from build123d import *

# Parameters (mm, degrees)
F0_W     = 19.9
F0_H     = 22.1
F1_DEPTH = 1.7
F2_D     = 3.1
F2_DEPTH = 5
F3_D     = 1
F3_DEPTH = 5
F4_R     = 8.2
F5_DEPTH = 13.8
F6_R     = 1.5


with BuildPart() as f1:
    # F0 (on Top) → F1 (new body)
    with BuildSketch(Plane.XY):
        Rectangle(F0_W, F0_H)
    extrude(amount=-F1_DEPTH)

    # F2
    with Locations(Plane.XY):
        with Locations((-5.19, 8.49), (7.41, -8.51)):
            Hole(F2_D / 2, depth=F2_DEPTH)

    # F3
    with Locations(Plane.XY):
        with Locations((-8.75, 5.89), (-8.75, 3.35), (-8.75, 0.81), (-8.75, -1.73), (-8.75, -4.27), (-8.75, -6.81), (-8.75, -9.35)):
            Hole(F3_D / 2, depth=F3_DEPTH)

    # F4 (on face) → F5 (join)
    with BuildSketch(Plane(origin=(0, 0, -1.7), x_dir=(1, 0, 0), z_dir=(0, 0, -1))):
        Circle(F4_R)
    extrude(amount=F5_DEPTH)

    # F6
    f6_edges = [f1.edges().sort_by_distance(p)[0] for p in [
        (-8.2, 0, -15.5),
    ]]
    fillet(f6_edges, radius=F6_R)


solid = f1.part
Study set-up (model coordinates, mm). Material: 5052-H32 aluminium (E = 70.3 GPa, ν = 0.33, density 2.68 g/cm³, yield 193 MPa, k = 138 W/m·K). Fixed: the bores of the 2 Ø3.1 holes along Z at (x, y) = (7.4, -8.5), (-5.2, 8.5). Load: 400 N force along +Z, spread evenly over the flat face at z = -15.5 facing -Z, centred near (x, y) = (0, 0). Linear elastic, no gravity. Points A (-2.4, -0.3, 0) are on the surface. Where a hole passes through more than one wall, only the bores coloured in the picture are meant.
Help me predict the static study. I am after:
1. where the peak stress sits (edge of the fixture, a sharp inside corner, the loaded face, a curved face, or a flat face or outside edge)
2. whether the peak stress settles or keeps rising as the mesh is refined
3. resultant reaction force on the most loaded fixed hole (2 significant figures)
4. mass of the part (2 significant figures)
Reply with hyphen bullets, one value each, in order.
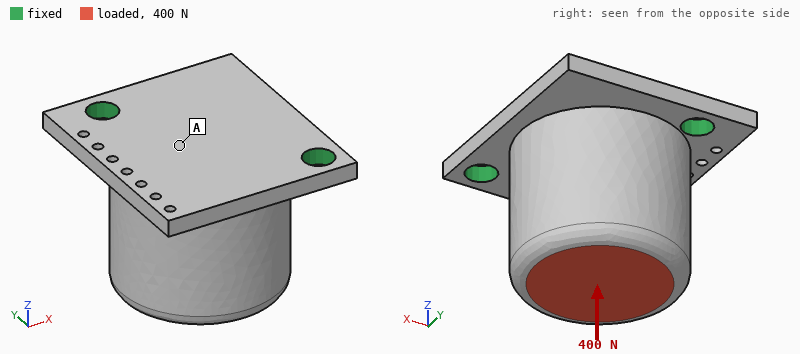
- edge of the fixture
- keeps rising
- 230 N
- 9.7 g
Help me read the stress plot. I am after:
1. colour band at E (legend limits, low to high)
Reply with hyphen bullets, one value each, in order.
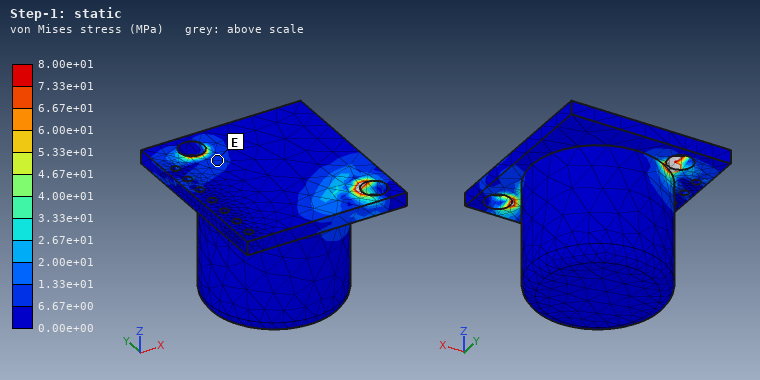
- 6.67e+00 to 1.33e+01 MPa
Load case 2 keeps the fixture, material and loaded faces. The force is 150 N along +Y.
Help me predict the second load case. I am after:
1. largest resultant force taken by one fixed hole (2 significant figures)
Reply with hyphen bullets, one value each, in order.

- 130 N
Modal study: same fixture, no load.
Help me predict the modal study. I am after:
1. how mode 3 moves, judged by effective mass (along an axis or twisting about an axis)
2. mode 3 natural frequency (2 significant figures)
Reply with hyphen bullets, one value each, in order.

- along Z
- 21 kHz
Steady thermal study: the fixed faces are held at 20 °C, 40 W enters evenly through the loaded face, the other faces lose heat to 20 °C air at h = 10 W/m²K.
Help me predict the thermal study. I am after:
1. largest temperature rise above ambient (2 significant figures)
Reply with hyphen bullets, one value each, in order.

- 53 K
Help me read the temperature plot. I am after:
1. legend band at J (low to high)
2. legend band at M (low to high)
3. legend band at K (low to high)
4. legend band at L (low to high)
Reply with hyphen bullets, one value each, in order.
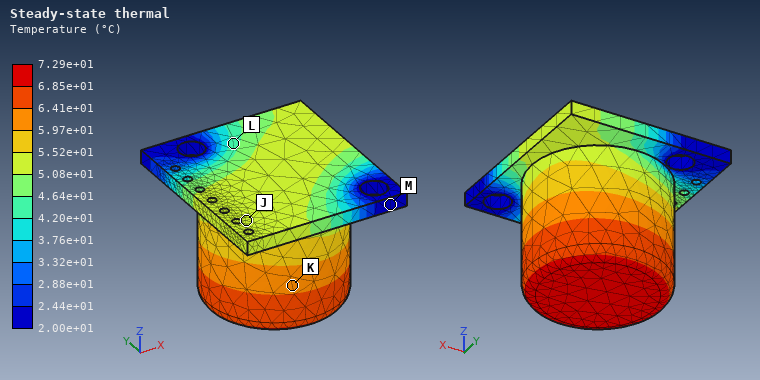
- 5.08e+01 to 5.52e+01 °C
- 2.00e+01 to 2.44e+01 °C
- 5.97e+01 to 6.41e+01 °C
- 4.20e+01 to 4.64e+01 °C
